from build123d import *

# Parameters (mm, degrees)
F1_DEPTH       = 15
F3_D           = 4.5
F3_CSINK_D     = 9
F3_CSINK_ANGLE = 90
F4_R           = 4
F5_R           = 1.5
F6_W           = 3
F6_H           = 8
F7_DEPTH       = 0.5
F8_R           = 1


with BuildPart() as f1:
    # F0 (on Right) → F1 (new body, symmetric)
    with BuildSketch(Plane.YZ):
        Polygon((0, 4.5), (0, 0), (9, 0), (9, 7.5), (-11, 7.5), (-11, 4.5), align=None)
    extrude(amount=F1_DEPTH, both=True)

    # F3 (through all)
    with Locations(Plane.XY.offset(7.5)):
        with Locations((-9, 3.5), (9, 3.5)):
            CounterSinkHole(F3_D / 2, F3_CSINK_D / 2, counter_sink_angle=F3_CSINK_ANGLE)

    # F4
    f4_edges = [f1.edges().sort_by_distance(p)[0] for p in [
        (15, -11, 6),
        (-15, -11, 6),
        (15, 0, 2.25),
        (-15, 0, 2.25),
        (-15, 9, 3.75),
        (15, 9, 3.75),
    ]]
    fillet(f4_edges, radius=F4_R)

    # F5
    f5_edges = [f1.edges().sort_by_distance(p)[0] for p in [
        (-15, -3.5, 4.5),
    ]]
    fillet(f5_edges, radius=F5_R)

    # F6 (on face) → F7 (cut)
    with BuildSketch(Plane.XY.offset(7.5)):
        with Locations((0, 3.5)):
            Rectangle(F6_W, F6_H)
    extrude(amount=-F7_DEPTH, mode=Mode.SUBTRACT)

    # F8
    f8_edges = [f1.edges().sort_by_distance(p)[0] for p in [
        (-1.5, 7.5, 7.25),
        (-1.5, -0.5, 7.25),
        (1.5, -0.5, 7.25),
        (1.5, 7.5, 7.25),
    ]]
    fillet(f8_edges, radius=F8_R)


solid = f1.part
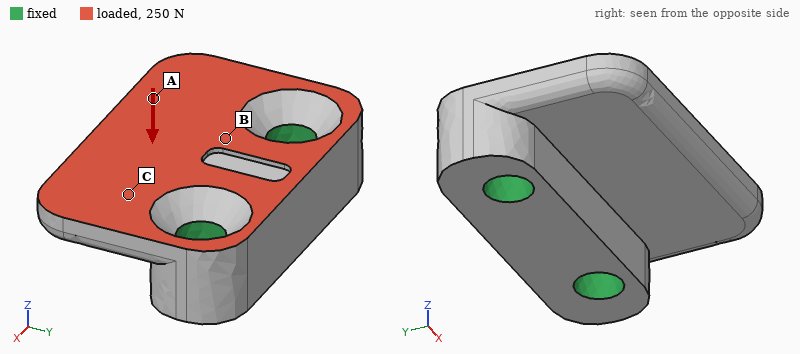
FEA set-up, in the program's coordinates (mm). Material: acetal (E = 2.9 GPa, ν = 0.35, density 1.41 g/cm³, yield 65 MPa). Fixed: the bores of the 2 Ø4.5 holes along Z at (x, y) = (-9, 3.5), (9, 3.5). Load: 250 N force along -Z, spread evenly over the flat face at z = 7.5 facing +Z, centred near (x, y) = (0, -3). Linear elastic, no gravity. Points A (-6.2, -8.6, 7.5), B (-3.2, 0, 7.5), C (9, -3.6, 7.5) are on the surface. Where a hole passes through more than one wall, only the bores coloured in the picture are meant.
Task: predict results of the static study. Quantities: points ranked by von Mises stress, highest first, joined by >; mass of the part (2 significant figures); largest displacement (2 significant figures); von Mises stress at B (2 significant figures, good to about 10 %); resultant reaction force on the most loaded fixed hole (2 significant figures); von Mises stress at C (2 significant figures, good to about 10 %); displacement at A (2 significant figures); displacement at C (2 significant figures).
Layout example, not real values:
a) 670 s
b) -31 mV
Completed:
a) B > C > A
b) 3.6 g
c) 0.39 mm
d) 23 MPa
e) 130 N
f) 7.3 MPa
g) 0.31 mm
h) 0.14 mm
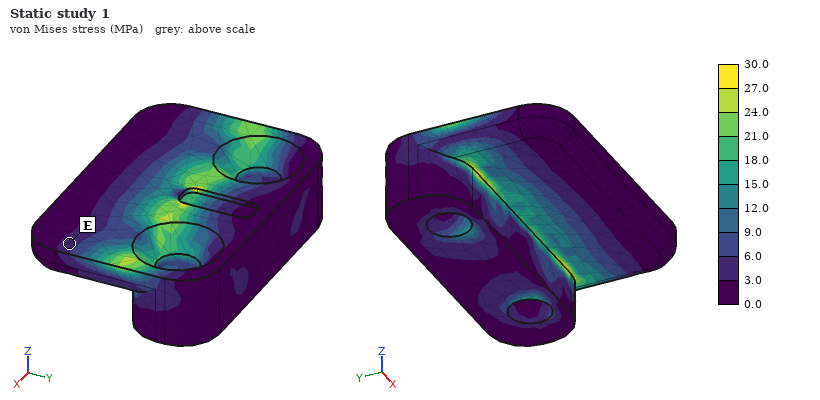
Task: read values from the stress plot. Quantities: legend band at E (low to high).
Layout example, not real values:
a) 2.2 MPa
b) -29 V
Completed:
a) 3.0 to 6.0 MPa
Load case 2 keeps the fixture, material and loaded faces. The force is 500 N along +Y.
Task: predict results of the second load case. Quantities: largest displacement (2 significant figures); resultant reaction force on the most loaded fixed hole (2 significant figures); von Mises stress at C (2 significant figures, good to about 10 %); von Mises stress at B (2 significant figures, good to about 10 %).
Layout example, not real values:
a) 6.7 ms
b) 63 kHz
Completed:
a) 0.33 mm
b) 250 N
c) 8.6 MPa
d) 18 MPa
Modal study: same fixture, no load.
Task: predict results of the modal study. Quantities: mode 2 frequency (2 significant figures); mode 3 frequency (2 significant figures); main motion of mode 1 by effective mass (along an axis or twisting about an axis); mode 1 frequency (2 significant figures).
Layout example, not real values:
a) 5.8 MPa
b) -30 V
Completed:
a) 5400 Hz
b) 9400 Hz
c) along Z
d) 3700 Hz
